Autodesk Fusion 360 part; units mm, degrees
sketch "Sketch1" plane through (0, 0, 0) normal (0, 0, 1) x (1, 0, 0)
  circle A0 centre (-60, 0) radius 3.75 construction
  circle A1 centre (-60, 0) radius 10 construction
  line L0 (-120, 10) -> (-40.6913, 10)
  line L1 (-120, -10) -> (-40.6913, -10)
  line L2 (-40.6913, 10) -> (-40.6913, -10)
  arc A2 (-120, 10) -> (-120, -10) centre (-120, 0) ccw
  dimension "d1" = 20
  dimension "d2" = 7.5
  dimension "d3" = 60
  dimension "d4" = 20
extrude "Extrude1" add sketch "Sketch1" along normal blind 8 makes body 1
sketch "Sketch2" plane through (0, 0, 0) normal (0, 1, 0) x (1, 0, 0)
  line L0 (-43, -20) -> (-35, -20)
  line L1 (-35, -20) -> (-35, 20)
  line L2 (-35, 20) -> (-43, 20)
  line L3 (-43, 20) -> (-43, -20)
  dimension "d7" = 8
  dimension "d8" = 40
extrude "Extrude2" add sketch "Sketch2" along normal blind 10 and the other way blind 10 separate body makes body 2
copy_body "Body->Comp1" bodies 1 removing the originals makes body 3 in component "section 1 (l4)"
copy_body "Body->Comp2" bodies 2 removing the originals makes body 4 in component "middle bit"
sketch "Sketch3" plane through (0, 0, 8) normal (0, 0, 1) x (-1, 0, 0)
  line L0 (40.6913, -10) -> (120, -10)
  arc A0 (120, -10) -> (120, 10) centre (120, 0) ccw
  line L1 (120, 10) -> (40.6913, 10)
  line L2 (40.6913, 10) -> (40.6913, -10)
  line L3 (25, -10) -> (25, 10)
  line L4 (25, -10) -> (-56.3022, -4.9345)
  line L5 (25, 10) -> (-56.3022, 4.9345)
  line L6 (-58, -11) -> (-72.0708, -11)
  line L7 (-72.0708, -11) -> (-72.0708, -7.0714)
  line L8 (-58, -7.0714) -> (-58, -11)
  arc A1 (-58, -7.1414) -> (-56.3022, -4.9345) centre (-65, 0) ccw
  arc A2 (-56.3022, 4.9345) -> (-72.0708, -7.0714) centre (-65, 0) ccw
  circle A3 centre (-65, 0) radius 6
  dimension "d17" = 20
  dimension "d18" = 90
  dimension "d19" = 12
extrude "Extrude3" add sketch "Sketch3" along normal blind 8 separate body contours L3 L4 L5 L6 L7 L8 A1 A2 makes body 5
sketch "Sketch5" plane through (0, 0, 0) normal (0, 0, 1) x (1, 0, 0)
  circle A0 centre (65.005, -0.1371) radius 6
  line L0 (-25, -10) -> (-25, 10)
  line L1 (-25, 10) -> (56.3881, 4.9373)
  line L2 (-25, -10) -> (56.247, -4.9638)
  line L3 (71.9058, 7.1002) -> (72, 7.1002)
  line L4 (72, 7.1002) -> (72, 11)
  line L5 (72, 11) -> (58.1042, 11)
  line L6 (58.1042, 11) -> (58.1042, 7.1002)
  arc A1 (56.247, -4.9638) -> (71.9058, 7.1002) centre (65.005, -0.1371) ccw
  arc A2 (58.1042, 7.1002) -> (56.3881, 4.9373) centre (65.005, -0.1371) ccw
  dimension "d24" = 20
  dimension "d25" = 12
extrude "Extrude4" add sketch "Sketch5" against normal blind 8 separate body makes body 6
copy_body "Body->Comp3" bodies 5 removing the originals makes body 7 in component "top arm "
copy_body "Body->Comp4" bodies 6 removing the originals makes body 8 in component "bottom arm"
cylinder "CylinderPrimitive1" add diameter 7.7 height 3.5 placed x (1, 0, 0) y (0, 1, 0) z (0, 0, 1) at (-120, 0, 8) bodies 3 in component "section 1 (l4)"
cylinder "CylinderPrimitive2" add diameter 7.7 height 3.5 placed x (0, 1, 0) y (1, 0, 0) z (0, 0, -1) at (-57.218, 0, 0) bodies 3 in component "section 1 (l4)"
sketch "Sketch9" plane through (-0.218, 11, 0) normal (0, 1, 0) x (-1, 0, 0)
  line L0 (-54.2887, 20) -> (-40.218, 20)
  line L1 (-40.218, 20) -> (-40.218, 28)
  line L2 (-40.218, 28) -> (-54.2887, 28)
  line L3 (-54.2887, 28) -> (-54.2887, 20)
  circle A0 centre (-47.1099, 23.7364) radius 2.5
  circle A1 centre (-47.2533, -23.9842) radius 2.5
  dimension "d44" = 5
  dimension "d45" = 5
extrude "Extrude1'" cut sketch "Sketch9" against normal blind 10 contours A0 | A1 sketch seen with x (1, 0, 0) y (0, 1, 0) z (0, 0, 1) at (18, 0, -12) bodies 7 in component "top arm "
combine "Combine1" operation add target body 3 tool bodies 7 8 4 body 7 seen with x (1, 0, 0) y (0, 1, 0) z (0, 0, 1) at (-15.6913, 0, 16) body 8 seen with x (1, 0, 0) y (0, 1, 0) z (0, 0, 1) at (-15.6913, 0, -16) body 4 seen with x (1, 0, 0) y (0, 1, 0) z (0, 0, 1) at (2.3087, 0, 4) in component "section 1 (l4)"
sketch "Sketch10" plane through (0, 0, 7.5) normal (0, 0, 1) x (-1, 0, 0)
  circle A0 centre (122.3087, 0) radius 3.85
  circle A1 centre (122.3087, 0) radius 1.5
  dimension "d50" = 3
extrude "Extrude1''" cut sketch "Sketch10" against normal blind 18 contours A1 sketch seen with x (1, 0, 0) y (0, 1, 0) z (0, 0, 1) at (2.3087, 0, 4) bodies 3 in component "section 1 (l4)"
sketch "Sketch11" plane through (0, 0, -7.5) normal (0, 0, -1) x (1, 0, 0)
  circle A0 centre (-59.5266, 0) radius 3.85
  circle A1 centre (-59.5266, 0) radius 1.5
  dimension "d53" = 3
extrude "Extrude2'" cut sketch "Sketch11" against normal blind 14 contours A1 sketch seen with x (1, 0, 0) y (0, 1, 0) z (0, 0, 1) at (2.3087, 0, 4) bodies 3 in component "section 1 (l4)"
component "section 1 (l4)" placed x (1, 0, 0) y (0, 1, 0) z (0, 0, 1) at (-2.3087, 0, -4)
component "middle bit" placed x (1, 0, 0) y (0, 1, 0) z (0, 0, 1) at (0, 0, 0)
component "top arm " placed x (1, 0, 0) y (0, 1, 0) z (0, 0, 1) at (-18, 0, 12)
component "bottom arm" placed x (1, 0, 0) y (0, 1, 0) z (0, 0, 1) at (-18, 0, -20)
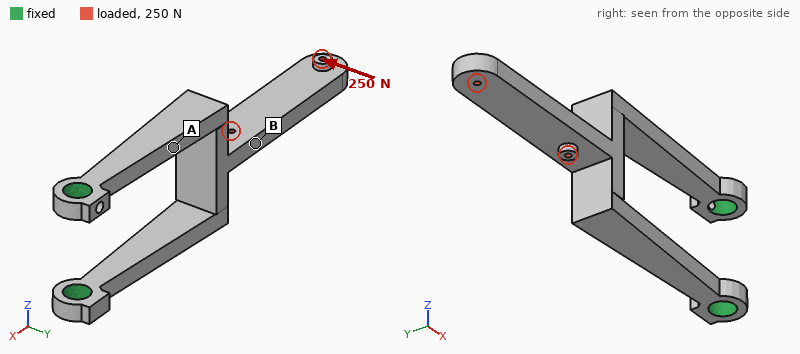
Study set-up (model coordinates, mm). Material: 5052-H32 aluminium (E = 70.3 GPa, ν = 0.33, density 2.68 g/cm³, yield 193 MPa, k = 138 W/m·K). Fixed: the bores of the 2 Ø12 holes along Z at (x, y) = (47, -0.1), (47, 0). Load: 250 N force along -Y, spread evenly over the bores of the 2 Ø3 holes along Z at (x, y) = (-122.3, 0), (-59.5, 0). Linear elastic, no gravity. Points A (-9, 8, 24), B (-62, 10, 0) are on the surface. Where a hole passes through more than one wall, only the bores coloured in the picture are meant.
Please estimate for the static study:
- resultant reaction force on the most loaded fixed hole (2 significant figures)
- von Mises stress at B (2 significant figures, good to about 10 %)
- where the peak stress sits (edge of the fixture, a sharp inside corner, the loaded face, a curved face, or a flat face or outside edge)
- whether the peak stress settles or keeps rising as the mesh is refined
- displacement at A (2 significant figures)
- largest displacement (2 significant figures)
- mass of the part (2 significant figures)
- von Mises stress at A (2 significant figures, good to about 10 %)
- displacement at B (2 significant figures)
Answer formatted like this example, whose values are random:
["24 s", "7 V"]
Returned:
["130 N", "14 MPa", "a sharp inside corner", "keeps rising", "0.28 mm", "1.6 mm", "120 g", "31 MPa", "0.81 mm"]
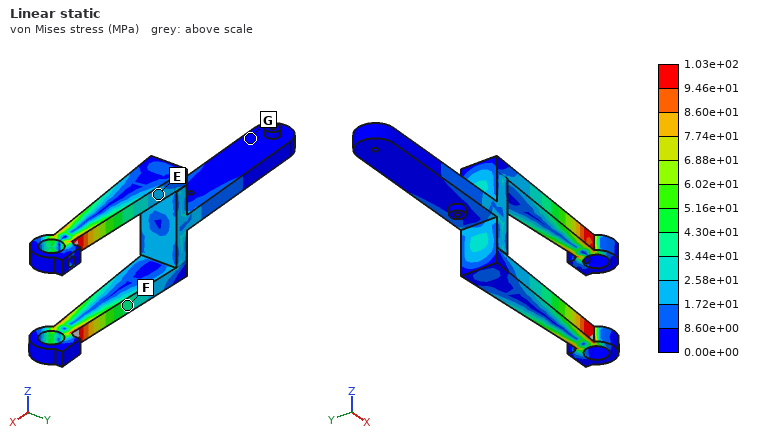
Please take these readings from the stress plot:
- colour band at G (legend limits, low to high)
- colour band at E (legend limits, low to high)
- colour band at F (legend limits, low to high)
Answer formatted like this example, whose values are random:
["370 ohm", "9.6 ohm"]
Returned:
["0.00e+00 to 8.60e+00 MPa", "1.72e+01 to 2.58e+01 MPa", "3.44e+01 to 4.30e+01 MPa"]
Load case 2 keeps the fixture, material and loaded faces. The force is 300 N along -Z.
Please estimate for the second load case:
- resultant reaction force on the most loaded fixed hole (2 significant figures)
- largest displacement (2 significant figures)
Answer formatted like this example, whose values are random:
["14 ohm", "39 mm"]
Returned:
["620 N", "0.79 mm"]
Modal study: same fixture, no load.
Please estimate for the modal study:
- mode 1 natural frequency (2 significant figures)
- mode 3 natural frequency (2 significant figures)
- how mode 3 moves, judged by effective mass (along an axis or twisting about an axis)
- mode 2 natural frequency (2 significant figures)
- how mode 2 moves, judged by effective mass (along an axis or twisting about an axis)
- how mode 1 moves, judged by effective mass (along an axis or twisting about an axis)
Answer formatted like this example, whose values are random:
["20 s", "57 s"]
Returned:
["350 Hz", "1100 Hz", "along Z", "610 Hz", "along Z", "along Y"]
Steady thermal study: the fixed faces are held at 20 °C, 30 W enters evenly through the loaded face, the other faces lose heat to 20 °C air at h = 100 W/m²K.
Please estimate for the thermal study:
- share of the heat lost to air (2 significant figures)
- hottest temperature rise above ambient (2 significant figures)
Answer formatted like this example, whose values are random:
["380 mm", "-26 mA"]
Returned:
["87 %", "49 K"]
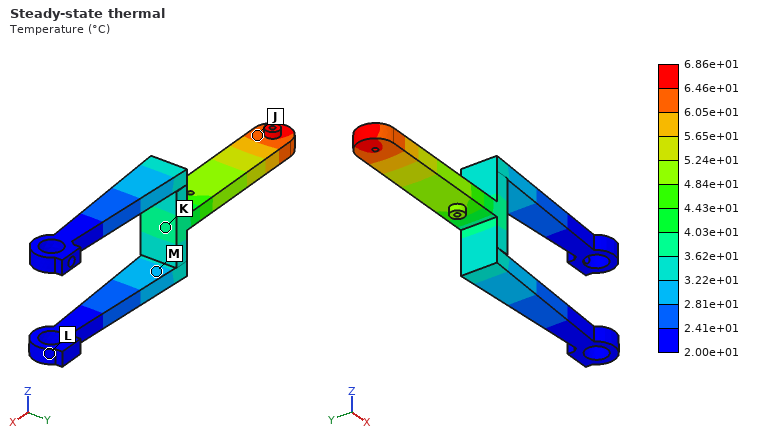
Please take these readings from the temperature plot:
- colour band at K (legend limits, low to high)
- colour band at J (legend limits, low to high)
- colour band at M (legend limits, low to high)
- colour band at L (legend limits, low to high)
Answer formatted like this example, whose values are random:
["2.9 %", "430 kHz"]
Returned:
["3.62e+01 to 4.03e+01 °C", "6.05e+01 to 6.46e+01 °C", "2.81e+01 to 3.22e+01 °C", "2.00e+01 to 2.41e+01 °C"]
